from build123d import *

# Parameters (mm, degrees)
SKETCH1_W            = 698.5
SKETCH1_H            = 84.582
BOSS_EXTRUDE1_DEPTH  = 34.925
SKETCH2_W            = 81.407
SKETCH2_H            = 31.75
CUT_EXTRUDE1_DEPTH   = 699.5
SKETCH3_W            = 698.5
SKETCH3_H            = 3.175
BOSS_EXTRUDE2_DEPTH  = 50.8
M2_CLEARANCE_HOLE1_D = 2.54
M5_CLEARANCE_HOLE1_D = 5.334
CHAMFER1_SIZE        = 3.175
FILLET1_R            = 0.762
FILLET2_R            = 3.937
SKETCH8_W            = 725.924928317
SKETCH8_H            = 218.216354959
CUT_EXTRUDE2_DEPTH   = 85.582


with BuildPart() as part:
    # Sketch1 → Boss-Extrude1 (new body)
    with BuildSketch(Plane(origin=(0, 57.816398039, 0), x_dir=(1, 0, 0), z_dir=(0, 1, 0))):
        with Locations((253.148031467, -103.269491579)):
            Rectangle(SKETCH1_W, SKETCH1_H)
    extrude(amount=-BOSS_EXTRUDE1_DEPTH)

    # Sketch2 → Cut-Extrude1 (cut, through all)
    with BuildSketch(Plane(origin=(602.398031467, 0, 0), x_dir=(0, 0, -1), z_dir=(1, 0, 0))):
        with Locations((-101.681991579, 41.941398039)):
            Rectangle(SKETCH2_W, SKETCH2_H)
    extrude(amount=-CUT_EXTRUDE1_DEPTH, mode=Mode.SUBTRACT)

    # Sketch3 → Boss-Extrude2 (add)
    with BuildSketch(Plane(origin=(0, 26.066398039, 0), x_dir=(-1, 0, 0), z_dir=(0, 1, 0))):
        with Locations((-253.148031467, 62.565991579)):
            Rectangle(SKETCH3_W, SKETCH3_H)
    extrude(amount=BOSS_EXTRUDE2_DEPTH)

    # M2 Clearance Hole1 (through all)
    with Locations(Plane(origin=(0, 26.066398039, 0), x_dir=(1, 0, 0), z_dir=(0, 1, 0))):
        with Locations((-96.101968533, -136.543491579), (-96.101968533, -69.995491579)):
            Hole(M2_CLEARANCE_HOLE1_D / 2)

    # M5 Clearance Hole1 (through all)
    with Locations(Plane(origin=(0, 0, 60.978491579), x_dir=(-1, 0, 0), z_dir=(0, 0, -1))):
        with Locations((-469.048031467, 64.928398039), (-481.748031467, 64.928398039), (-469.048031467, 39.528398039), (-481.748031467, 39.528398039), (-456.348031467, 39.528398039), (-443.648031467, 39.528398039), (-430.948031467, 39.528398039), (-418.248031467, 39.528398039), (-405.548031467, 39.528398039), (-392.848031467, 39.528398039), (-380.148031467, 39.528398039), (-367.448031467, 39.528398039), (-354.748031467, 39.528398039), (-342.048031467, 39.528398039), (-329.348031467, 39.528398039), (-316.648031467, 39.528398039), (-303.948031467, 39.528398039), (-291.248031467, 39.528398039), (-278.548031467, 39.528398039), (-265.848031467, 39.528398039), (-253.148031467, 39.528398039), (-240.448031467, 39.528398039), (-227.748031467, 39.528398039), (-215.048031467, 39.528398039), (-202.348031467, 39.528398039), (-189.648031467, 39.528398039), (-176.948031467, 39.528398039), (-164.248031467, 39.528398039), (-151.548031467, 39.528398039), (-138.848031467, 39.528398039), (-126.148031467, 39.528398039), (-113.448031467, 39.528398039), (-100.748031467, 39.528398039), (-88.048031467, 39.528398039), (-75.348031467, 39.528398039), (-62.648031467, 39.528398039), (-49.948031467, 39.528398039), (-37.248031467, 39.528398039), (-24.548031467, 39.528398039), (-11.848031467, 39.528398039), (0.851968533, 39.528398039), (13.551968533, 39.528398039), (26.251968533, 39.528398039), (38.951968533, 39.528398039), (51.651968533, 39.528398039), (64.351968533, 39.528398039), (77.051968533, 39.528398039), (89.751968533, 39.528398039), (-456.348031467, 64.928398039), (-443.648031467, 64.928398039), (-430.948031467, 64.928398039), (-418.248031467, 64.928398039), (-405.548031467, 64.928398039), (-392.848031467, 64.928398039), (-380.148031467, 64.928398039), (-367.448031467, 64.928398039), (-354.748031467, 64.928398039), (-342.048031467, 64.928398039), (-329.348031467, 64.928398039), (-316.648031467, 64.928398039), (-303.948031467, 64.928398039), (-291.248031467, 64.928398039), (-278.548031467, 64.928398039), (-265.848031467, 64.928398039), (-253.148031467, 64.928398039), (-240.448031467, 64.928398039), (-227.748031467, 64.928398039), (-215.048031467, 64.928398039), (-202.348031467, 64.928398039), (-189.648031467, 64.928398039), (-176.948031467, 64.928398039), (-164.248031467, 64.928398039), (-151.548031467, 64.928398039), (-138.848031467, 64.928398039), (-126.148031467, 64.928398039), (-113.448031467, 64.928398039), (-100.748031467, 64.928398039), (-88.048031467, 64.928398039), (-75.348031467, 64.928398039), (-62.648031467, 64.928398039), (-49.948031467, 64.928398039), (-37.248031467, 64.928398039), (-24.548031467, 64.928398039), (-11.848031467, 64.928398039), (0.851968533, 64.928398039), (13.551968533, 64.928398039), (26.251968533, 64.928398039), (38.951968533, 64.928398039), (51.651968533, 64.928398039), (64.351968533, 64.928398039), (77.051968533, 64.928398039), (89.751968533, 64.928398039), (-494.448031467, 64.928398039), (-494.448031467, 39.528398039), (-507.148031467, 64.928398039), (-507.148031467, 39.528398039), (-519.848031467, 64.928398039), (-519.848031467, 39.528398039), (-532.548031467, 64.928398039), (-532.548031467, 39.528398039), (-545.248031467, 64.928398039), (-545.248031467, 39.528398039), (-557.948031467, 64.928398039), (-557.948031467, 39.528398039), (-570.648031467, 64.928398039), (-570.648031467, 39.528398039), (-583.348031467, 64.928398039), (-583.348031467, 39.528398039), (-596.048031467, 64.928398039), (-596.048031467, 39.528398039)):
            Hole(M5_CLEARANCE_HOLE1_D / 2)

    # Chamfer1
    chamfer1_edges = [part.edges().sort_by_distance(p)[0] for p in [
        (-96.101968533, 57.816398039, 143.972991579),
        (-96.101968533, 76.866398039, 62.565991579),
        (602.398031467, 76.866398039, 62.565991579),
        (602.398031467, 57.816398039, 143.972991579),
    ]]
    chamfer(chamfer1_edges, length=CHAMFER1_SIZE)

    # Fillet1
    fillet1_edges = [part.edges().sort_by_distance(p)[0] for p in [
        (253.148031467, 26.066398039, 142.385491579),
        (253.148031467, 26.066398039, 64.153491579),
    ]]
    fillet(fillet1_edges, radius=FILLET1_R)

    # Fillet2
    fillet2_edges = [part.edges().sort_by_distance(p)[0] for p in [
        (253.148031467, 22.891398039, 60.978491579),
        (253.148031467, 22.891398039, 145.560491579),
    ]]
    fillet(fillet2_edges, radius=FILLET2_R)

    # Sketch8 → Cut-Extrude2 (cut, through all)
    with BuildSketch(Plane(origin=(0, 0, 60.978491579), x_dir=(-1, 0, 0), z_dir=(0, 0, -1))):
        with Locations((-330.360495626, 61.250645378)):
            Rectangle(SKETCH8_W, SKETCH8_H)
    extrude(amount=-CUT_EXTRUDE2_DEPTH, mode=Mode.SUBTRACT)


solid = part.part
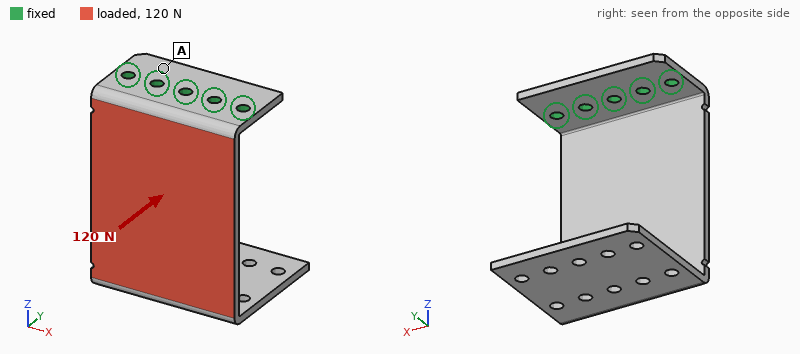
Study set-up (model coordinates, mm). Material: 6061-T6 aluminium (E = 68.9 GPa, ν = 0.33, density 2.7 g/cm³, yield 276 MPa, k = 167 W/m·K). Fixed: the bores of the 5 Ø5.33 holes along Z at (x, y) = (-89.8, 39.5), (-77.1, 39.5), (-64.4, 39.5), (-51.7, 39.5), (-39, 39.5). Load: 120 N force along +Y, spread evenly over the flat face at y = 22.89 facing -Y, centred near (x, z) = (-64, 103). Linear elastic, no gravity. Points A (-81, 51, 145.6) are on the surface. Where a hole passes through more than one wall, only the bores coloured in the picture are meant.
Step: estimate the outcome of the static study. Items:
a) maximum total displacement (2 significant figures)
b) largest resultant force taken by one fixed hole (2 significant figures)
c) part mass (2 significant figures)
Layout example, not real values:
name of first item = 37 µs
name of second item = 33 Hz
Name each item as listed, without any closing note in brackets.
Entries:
maximum total displacement = 1.3 mm
largest resultant force taken by one fixed hole = 39 N
part mass = 87 g
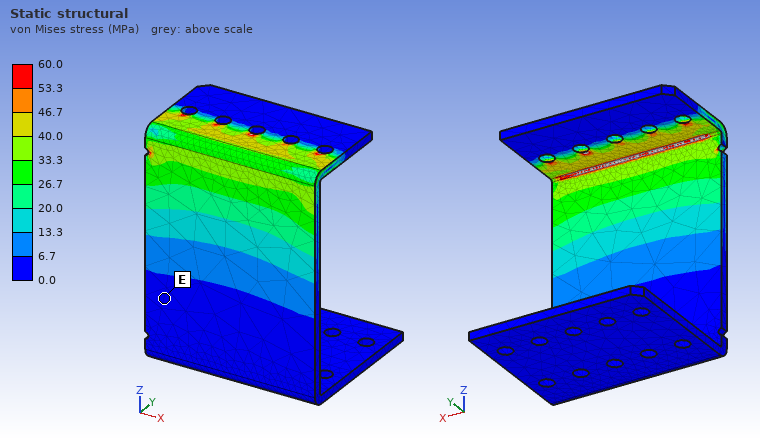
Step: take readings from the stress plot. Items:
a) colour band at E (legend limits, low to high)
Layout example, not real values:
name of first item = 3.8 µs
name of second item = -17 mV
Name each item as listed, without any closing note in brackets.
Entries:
colour band at E = 0.0 to 6.7 MPa
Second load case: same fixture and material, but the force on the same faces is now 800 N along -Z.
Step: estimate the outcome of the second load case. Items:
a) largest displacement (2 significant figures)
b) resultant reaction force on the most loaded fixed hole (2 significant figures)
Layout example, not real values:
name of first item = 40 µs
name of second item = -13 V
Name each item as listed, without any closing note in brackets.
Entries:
largest displacement = 0.96 mm
resultant reaction force on the most loaded fixed hole = 160 N
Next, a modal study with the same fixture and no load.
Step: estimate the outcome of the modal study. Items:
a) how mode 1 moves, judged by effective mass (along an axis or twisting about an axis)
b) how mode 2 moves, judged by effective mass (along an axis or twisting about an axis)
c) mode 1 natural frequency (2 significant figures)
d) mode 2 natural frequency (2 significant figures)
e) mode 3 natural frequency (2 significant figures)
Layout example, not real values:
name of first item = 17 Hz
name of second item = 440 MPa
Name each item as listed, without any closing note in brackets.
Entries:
how mode 1 moves, judged by effective mass = along Y
how mode 2 moves, judged by effective mass = along X
mode 1 natural frequency = 170 Hz
mode 2 natural frequency = 380 Hz
mode 3 natural frequency = 590 Hz
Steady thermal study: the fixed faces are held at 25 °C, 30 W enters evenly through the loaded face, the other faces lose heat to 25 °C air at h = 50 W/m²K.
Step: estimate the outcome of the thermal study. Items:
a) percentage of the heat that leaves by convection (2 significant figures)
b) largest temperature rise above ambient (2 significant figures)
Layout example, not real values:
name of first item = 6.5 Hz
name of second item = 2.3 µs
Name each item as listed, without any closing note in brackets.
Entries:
percentage of the heat that leaves by convection = 40 %
largest temperature rise above ambient = 23 K
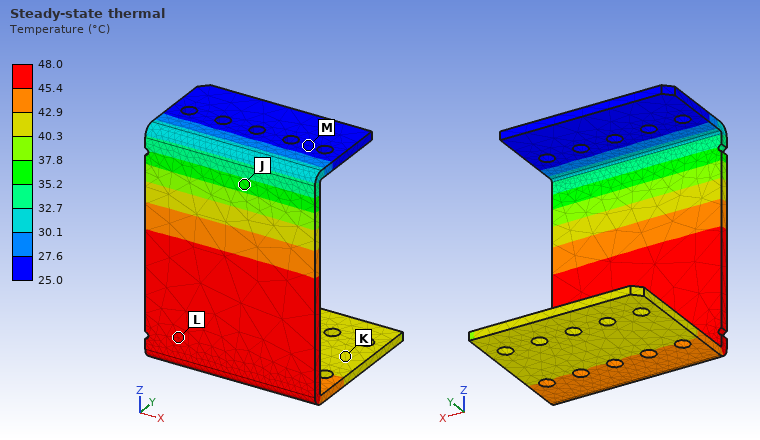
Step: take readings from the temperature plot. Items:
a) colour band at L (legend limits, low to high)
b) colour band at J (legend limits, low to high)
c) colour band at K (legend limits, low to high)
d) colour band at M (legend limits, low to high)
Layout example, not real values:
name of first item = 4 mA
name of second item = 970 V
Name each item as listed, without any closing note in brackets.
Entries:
colour band at L = 45.4 to 48.0 °C
colour band at J = 35.2 to 37.8 °C
colour band at K = 40.3 to 42.9 °C
colour band at M = 25.0 to 27.6 °C
